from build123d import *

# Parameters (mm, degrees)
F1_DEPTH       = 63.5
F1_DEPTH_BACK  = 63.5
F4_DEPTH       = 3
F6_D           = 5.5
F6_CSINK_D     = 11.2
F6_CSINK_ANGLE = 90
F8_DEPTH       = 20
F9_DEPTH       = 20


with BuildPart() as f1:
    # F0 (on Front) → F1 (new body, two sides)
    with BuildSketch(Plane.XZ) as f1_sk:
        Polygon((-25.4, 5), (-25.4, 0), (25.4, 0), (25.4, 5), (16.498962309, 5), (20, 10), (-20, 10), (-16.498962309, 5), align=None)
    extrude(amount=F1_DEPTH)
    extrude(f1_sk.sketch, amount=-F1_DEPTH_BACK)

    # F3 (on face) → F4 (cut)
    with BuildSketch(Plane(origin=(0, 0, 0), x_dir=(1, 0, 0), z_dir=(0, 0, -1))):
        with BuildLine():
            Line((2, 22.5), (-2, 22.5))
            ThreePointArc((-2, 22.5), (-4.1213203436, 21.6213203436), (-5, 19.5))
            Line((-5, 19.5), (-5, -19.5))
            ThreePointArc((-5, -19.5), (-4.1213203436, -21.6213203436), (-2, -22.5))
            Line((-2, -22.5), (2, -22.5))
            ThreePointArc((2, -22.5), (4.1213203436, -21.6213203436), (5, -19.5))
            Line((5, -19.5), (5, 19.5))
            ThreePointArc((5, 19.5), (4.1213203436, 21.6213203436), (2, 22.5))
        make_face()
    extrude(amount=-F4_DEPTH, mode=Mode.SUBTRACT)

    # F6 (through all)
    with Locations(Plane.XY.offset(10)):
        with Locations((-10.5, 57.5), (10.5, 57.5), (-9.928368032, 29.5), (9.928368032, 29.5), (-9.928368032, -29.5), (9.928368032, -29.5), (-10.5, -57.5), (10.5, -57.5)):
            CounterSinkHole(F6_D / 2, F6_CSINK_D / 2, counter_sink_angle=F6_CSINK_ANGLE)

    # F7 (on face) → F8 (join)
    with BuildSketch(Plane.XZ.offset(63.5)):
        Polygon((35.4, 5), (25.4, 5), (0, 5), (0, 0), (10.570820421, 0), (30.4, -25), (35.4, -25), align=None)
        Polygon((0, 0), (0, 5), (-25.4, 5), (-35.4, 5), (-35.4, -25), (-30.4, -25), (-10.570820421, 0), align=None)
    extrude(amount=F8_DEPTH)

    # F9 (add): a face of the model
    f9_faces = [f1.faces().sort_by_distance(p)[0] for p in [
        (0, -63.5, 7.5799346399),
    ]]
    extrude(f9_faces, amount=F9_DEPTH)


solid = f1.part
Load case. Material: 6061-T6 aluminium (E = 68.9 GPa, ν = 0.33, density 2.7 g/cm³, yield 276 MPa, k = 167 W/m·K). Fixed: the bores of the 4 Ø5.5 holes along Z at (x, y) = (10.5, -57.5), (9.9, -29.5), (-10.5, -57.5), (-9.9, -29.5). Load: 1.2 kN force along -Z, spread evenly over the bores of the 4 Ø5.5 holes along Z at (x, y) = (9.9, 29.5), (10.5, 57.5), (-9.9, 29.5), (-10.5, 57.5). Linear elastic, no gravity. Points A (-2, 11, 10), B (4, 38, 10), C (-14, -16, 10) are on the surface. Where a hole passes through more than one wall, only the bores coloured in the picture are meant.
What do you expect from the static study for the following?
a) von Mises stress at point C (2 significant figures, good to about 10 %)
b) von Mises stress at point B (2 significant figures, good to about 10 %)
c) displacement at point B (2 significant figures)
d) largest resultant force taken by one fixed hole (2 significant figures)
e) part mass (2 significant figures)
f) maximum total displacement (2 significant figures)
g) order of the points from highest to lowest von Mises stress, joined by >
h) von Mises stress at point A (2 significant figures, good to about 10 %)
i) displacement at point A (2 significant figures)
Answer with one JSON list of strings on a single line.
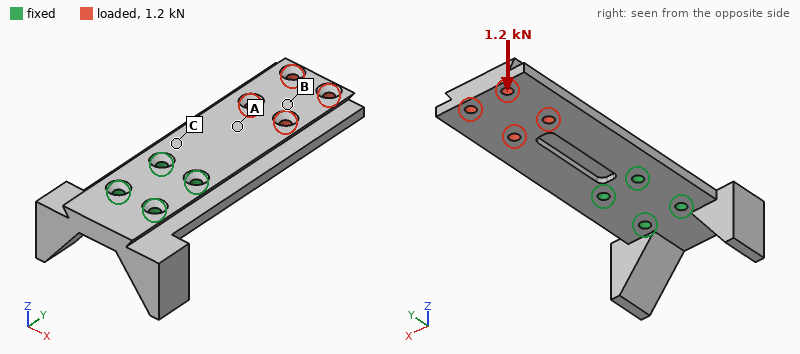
["110 MPa", "24 MPa", "0.69 mm", "1.1 kN", "210 g", "1.1 mm", "C > A > B", "59 MPa", "0.31 mm"]
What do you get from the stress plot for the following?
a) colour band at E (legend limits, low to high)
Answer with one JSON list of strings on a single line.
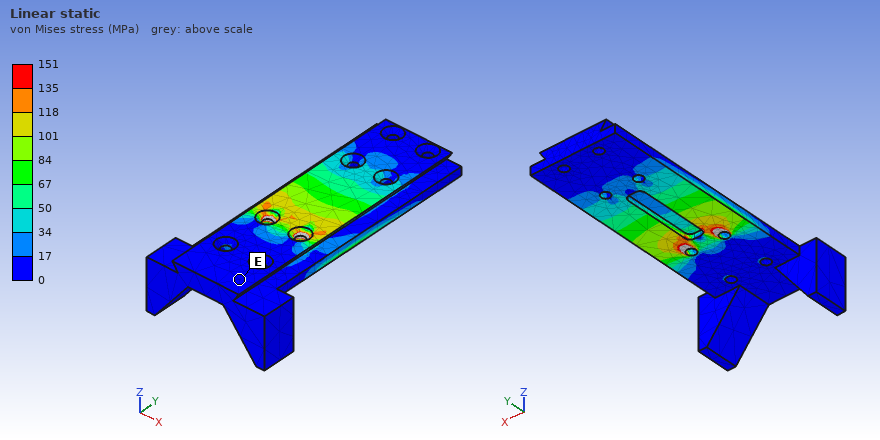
["0 to 17 MPa"]
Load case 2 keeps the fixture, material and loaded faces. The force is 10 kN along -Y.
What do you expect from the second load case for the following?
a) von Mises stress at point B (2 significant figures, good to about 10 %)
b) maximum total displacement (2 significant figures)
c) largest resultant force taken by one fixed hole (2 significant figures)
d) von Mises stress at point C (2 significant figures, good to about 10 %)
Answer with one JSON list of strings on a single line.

["7.5 MPa", "0.23 mm", "4.3 kN", "6.1 MPa"]
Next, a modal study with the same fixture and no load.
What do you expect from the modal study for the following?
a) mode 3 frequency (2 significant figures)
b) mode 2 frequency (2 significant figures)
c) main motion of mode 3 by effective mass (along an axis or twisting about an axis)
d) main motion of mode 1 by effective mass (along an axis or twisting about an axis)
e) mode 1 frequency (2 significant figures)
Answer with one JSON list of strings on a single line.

["3400 Hz", "2800 Hz", "along X", "along Z", "880 Hz"]
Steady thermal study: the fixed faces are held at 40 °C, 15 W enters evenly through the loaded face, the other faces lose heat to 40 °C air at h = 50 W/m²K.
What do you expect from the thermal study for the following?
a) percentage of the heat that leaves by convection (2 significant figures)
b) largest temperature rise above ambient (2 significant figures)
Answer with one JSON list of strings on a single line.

["31 %", "13 K"]
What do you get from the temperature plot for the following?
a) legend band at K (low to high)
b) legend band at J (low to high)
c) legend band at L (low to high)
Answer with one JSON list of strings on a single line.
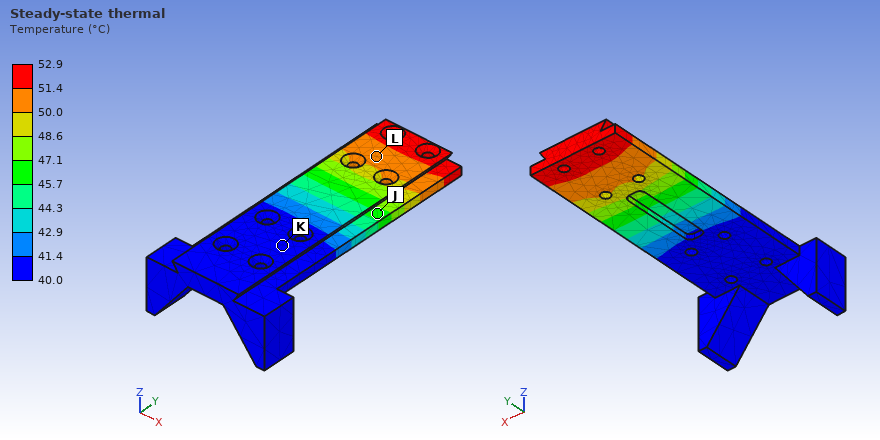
["40.0 to 41.4 °C", "45.7 to 47.1 °C", "50.0 to 51.4 °C"]
